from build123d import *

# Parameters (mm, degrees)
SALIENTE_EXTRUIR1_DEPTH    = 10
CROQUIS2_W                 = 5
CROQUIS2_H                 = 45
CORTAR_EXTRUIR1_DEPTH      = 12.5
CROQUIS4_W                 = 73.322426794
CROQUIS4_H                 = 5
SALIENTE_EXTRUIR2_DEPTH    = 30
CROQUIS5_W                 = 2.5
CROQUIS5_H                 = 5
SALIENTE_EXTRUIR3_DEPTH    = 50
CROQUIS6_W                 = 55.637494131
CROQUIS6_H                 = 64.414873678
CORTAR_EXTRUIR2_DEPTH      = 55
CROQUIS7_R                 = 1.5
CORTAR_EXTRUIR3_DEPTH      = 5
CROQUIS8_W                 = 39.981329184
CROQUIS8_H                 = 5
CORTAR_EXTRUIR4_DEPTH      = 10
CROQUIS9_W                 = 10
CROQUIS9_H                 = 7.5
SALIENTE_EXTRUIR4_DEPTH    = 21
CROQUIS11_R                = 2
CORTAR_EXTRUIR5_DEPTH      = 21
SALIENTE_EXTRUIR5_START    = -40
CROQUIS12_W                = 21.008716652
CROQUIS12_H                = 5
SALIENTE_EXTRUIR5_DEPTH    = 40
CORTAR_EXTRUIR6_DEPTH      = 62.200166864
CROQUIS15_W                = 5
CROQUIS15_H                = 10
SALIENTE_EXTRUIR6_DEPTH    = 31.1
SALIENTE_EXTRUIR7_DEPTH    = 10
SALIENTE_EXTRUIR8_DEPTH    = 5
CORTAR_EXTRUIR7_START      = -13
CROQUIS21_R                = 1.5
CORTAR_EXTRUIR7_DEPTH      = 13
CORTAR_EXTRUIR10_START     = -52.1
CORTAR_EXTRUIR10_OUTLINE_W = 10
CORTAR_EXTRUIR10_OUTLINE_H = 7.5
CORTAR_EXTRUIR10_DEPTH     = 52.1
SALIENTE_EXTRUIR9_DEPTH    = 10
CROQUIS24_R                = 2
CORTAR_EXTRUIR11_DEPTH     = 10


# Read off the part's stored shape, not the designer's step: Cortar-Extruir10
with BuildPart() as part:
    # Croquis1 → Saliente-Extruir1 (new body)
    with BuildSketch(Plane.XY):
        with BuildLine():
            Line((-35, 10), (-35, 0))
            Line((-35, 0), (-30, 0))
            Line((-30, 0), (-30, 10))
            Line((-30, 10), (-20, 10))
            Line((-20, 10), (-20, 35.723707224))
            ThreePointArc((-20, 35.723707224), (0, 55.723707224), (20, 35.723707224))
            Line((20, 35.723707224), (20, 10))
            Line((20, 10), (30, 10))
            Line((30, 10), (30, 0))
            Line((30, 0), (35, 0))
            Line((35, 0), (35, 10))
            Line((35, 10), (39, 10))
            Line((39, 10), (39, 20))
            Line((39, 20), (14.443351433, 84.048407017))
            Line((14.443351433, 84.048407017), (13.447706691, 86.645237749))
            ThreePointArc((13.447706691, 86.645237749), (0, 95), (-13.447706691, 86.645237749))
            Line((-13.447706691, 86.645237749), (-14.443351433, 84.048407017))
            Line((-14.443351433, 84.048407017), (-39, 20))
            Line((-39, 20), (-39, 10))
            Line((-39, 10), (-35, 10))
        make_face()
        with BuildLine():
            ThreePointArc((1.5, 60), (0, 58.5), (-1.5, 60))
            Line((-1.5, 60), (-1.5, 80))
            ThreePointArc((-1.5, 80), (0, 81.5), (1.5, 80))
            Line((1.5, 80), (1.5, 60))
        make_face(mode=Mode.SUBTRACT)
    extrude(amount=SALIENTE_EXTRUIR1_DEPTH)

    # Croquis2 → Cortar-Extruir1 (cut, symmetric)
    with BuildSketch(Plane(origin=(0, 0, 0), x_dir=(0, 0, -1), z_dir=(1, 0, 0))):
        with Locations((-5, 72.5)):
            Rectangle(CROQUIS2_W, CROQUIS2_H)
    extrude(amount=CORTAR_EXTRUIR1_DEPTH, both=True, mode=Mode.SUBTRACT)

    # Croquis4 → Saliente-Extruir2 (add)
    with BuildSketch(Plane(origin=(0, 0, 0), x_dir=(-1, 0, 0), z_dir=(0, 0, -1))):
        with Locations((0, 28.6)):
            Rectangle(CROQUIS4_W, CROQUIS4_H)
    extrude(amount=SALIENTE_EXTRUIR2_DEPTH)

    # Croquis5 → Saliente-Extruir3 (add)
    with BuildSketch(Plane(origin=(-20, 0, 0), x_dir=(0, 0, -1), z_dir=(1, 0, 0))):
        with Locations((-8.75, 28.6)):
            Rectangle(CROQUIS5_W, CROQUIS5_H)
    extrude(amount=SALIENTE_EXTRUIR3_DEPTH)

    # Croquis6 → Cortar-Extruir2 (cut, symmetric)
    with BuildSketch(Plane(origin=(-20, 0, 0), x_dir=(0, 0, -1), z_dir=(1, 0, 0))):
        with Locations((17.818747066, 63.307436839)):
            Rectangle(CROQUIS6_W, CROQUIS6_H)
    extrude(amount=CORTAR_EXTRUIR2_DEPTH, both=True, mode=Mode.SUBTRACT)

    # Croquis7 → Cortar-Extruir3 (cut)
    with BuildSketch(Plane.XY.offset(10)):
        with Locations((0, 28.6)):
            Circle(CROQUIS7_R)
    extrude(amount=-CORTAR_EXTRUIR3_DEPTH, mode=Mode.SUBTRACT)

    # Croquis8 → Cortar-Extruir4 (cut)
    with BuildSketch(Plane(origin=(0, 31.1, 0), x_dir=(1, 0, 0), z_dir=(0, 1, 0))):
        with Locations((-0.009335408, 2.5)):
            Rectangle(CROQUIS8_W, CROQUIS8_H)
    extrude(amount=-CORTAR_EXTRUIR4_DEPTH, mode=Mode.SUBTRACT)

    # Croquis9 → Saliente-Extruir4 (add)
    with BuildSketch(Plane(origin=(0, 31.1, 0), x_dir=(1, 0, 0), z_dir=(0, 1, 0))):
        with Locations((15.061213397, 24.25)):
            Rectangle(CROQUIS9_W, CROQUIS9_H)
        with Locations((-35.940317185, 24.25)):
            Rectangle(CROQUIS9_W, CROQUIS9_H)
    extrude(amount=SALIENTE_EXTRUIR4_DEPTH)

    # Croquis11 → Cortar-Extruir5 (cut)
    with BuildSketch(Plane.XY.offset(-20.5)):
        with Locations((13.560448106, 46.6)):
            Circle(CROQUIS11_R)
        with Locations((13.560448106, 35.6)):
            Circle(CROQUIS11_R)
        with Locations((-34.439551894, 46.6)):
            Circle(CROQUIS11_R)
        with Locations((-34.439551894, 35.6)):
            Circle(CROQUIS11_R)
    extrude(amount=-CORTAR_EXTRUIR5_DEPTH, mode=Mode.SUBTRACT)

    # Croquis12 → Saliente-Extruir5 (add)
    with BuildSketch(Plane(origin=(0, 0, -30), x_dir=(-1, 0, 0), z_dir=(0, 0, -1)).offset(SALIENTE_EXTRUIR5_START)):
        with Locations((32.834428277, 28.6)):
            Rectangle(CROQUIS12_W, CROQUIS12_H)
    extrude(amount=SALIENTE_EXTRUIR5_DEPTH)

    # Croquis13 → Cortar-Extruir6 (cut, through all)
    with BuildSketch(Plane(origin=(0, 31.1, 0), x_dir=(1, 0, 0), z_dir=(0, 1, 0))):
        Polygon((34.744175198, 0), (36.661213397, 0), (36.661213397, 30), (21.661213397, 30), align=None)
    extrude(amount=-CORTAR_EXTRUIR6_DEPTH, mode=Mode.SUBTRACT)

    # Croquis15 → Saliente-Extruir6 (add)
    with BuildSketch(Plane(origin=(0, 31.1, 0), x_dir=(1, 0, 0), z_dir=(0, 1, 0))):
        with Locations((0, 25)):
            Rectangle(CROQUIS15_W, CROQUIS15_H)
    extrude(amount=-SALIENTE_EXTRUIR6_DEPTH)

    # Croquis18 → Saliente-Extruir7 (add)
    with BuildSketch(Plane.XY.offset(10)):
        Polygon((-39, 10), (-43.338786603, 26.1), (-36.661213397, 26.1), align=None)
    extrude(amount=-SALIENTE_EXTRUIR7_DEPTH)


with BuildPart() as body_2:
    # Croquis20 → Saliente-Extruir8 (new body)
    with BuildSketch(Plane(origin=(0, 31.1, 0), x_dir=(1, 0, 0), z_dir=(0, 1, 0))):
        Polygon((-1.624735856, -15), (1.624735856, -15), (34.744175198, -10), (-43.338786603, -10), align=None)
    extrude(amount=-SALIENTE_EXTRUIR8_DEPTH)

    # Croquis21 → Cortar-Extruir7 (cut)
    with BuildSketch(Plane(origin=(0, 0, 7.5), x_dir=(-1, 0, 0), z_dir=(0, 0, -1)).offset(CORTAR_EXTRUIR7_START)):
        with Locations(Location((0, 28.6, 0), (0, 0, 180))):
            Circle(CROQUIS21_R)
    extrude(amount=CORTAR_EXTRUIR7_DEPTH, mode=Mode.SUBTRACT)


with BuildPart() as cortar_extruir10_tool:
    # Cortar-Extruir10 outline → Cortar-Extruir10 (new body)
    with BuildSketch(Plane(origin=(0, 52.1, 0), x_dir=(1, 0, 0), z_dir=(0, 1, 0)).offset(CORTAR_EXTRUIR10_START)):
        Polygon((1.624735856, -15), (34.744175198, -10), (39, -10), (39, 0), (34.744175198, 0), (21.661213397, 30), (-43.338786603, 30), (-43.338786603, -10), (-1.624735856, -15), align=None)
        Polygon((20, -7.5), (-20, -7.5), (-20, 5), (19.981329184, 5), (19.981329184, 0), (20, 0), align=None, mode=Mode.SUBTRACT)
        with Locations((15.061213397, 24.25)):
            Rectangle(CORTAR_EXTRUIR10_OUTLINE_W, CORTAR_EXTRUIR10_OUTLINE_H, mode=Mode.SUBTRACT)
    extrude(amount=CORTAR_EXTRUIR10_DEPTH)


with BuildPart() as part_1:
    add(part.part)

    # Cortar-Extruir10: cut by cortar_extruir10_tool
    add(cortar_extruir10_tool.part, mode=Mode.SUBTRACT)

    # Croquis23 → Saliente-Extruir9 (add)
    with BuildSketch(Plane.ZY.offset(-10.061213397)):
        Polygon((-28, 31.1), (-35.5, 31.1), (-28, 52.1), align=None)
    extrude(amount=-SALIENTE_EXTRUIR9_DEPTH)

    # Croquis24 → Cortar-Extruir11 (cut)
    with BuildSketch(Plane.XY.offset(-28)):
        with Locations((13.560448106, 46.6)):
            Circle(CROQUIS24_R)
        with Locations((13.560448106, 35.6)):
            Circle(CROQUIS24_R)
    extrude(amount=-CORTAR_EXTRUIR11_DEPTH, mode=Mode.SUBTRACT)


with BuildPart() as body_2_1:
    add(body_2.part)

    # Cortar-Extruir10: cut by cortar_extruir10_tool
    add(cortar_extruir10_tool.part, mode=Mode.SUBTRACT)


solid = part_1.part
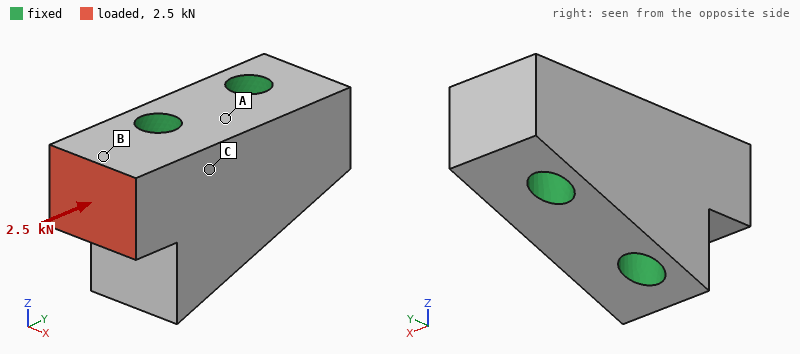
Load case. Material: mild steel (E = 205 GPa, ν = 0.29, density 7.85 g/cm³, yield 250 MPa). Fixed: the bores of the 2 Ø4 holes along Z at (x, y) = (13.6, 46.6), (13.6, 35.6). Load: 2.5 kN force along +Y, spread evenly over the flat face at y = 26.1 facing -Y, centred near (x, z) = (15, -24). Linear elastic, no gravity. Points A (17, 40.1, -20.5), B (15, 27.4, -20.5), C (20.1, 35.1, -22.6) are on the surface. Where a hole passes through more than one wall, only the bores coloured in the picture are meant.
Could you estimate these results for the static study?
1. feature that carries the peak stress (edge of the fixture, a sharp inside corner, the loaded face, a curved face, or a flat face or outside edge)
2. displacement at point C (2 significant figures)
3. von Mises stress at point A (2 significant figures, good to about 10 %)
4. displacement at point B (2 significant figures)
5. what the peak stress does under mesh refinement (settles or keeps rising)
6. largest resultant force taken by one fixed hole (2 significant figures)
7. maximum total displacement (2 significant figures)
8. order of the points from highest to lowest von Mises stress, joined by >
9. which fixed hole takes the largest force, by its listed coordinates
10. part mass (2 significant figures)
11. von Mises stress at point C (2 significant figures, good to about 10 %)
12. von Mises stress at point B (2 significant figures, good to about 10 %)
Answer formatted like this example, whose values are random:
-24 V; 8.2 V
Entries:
edge of the fixture; 0.78 µm; 11 MPa; 1.7 µm; keeps rising; 2.3 kN; 2.4 µm; B > C > A; (13.6, 35.6); 19 g; 25 MPa; 35 MPa
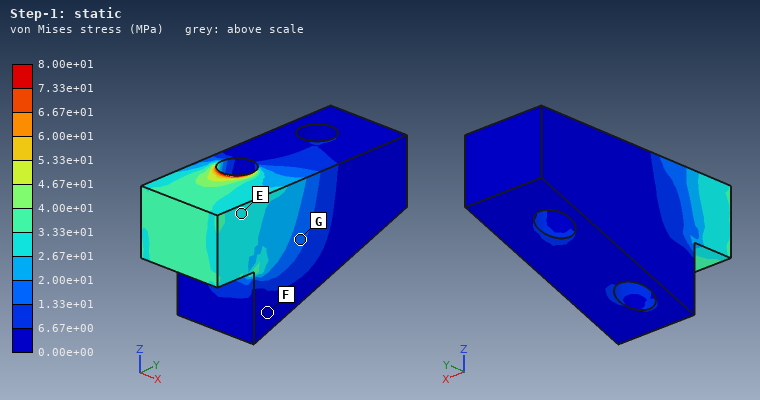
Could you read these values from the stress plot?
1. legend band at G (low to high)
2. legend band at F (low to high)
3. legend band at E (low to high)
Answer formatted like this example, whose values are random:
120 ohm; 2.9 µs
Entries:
1.33e+01 to 2.00e+01 MPa; 0.00e+00 to 6.67e+00 MPa; 2.67e+01 to 3.33e+01 MPa
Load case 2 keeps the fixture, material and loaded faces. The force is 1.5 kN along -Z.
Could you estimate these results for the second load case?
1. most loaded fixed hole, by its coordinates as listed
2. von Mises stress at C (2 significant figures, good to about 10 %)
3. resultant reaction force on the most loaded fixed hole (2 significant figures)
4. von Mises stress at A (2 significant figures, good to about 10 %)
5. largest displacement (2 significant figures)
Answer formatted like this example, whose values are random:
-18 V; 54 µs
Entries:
(13.6, 35.6); 23 MPa; 1.6 kN; 10 MPa; 6.3 µm
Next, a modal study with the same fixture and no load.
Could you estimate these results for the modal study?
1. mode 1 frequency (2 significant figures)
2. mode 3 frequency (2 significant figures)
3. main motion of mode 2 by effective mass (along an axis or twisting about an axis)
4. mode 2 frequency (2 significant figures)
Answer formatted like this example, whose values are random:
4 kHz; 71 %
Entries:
57 kHz; 93 kHz; along Z; 68 kHz
